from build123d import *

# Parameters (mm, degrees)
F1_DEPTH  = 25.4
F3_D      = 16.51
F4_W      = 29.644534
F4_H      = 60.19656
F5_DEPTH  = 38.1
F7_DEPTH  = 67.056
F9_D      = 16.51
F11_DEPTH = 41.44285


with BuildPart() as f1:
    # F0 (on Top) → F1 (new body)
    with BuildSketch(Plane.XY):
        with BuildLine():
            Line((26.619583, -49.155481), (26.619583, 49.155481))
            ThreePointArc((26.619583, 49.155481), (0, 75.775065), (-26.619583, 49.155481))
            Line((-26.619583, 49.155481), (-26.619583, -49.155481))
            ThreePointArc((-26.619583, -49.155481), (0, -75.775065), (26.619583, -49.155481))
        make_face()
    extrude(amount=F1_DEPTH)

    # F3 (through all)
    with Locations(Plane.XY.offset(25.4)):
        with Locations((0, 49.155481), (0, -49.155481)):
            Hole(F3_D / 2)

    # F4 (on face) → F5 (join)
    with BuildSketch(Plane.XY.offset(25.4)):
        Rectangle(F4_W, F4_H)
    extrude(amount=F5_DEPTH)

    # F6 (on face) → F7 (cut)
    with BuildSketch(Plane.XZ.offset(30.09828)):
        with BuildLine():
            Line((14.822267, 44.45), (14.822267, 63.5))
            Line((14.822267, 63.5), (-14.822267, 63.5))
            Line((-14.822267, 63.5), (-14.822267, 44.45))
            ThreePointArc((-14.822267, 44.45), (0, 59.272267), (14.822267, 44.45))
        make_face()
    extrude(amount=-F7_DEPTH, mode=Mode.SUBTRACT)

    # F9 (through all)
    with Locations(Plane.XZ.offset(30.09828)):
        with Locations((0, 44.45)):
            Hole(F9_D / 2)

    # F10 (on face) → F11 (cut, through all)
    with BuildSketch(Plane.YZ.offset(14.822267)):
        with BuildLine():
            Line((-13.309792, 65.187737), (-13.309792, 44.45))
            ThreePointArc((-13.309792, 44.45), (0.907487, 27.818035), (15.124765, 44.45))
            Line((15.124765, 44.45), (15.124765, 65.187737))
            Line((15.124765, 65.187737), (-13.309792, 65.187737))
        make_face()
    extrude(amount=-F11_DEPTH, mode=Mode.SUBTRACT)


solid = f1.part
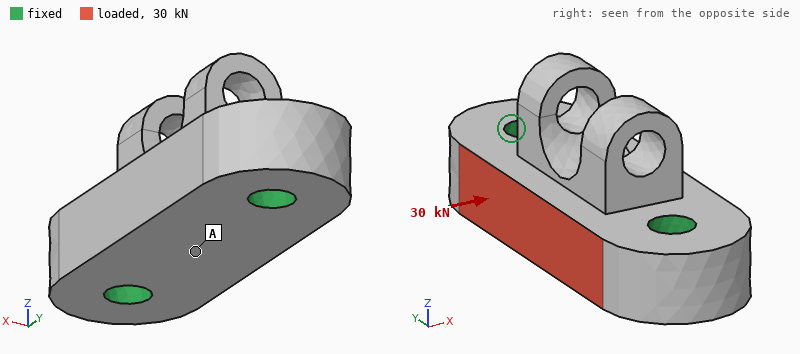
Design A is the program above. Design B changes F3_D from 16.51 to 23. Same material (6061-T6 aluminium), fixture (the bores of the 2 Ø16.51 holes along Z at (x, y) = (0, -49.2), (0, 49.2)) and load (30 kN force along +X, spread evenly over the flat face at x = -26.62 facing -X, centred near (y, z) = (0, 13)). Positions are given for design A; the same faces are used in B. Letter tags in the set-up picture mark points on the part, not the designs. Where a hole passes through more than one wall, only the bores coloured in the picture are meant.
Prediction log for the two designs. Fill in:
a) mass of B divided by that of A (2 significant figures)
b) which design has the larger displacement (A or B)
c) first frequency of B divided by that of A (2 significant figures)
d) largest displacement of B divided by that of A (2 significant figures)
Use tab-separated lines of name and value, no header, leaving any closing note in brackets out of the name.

mass of B divided by that of A	0.95
which design has the larger displacement	A
first frequency of B divided by that of A	1.1
largest displacement of B divided by that of A	0.81
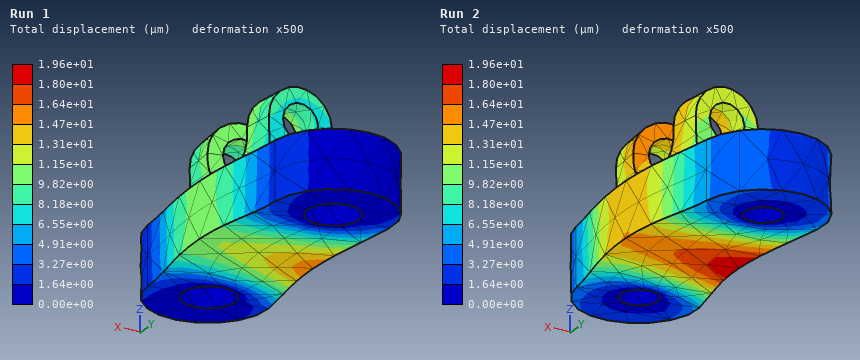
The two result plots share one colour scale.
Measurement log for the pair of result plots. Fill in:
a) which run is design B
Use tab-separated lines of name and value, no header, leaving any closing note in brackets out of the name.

which run is design B	Run 1
